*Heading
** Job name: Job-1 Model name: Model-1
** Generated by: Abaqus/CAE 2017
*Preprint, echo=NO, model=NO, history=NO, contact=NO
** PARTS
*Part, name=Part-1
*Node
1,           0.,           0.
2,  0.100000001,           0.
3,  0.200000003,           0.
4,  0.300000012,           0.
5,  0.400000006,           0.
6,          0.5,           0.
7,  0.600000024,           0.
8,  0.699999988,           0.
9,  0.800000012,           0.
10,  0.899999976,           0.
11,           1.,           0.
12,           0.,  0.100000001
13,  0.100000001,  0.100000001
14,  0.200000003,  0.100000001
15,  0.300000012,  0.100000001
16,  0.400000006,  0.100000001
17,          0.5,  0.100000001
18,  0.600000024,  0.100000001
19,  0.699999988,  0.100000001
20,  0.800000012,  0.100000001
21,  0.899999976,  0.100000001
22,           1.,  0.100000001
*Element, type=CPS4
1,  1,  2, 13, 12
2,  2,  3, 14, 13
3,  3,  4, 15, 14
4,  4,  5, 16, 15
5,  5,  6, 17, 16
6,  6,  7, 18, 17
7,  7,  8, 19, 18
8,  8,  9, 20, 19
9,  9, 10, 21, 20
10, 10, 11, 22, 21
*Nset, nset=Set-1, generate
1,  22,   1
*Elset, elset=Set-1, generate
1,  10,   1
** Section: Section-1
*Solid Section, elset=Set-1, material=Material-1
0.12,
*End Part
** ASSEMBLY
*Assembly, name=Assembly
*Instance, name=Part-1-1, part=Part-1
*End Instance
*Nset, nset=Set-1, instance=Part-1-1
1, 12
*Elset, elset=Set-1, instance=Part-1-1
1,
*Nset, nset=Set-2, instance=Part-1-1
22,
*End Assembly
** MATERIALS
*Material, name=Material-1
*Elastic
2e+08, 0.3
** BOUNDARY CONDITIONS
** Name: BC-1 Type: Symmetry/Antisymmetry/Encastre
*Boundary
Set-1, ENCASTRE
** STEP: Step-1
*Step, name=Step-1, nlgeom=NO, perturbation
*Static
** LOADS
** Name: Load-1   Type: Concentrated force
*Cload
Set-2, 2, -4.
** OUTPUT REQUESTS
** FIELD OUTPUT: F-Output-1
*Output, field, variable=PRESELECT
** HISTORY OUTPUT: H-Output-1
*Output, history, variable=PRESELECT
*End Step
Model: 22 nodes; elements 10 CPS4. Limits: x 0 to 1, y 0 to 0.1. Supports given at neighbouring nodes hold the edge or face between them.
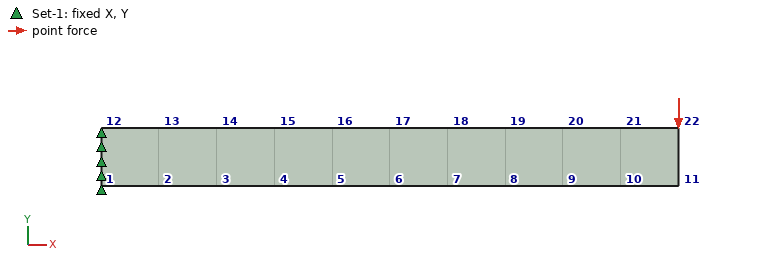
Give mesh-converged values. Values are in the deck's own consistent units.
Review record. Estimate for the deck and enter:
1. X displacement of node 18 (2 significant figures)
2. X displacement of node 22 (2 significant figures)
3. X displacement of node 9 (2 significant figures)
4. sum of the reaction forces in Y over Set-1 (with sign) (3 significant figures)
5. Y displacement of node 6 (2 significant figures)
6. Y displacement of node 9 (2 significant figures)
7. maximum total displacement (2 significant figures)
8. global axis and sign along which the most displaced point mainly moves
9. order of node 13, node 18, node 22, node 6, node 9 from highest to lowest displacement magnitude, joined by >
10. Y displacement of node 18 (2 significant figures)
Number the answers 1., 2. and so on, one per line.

1. 4.1e-05
2. 4.9e-05
3. -4.7e-05
4. 4.00
5. -2.0e-04
6. -4.6e-04
7. 6.5e-04
8. -Y
9. node 22 > node 9 > node 18 > node 6 > node 13
10. -2.8e-04
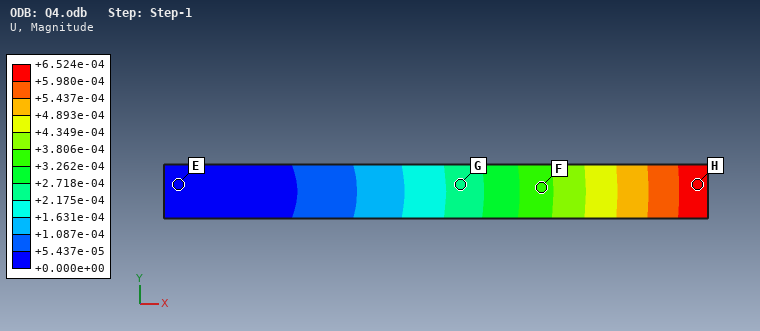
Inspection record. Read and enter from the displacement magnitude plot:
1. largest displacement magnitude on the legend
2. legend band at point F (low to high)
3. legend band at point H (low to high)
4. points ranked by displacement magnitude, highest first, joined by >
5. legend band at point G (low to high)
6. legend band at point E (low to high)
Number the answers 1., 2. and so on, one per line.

1. +6.524e-04
2. +3.262e-04 to +3.806e-04
3. +5.980e-04 to +6.524e-04
4. H > F > G > E
5. +2.175e-04 to +2.718e-04
6. +0.000e+00 to +5.437e-05
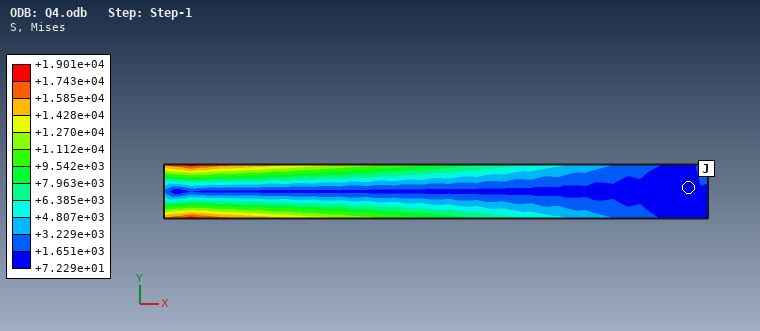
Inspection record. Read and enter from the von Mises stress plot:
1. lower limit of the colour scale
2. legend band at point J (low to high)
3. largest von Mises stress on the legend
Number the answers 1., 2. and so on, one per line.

1. +7.229e+01
2. +7.229e+01 to +1.651e+03
3. +1.901e+04
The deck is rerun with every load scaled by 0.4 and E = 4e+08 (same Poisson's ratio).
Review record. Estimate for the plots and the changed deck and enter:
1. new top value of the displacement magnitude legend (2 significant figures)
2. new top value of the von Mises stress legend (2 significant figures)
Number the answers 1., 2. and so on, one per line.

1. 1.3e-04
2. 7600
